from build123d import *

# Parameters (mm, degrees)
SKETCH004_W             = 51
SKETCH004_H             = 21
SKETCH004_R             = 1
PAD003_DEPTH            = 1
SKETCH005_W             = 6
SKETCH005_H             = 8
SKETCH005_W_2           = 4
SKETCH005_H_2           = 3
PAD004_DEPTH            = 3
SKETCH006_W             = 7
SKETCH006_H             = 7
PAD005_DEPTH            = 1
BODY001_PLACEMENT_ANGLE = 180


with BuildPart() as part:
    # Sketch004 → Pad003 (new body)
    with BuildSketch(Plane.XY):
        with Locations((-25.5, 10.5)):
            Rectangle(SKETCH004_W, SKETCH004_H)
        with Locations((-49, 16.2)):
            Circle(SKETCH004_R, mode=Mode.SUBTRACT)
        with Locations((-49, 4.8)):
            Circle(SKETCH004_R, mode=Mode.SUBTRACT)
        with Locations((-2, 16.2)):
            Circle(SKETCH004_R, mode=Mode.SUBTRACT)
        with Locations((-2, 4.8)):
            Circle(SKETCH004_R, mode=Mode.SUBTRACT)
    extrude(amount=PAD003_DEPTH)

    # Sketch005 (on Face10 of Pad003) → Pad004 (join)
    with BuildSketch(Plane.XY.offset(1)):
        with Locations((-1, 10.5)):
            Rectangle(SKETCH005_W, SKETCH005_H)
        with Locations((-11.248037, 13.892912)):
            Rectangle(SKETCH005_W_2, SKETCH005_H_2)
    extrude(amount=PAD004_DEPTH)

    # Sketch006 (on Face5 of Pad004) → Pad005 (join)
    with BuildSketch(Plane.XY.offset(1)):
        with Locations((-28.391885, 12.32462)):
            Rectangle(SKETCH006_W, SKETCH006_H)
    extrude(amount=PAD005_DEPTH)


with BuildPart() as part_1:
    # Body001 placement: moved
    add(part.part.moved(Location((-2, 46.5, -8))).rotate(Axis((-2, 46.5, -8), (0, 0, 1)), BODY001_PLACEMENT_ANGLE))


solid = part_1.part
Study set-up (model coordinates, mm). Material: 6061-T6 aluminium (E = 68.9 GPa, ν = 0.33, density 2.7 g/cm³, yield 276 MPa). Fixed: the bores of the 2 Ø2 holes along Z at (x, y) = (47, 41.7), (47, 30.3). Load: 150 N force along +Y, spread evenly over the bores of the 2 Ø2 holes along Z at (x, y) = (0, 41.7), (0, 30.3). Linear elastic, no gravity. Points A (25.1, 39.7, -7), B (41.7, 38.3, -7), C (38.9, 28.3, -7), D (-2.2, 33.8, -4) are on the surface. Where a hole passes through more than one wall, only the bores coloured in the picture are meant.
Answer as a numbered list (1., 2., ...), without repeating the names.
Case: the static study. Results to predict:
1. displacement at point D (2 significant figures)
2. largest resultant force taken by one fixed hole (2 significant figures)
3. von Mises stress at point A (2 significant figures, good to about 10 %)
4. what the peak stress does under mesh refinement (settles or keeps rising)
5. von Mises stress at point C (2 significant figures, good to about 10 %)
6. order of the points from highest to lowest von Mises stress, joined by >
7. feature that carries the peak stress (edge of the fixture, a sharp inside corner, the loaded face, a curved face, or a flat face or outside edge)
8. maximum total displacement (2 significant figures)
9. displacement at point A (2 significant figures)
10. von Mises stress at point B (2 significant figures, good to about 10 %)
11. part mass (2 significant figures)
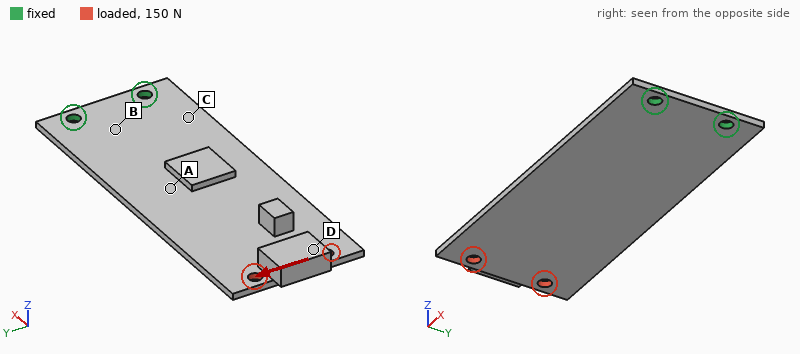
1. 0.14 mm
2. 560 N
3. 23 MPa
4. keeps rising
5. 60 MPa
6. C > B > A > D
7. edge of the fixture
8. 0.16 mm
9. 0.048 mm
10. 43 MPa
11. 3.5 g
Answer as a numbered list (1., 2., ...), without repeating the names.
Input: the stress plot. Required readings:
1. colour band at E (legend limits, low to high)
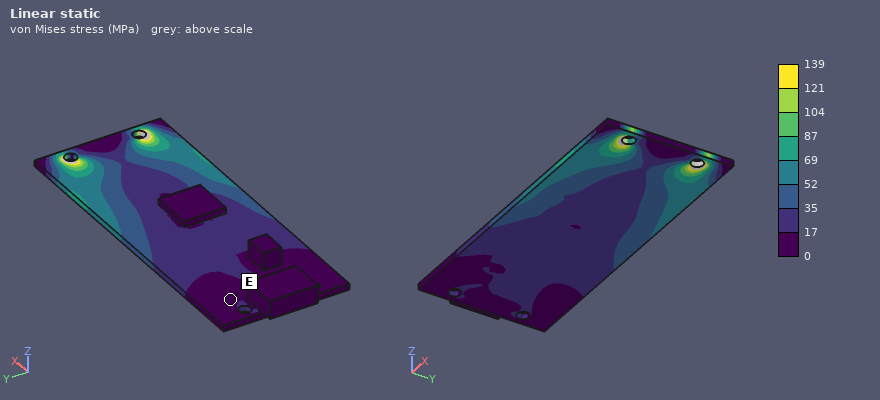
1. 0 to 17 MPa
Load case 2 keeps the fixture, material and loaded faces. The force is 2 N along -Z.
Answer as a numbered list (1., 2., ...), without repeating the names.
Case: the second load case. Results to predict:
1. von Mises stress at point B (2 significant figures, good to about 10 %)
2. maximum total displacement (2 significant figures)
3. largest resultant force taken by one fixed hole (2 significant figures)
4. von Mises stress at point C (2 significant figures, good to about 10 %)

1. 21 MPa
2. 0.58 mm
3. 1.1 N
4. 22 MPa
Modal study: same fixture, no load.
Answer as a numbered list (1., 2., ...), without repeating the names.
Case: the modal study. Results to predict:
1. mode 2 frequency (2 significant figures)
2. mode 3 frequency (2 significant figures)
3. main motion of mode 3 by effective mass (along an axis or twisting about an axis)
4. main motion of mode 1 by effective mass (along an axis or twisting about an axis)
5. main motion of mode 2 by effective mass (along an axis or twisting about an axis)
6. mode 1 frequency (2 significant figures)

1. 1800 Hz
2. 1900 Hz
3. along Z
4. along Z
5. twisting about X
6. 280 Hz
